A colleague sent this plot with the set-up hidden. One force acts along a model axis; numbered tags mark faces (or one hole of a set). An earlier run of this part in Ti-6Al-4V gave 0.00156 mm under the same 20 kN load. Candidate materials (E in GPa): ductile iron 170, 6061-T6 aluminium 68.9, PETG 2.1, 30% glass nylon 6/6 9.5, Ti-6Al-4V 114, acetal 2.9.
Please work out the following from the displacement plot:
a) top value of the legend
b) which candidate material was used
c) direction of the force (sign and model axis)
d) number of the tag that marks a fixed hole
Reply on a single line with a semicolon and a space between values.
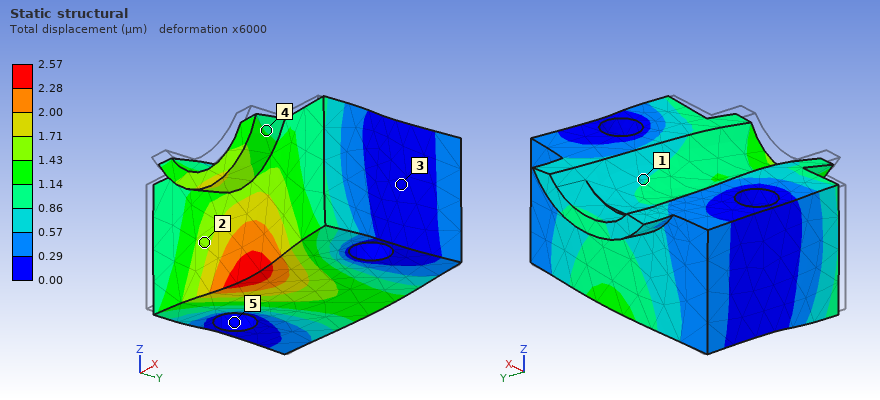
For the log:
2.57 µm; 6061-T6 aluminium; +Y; 5
